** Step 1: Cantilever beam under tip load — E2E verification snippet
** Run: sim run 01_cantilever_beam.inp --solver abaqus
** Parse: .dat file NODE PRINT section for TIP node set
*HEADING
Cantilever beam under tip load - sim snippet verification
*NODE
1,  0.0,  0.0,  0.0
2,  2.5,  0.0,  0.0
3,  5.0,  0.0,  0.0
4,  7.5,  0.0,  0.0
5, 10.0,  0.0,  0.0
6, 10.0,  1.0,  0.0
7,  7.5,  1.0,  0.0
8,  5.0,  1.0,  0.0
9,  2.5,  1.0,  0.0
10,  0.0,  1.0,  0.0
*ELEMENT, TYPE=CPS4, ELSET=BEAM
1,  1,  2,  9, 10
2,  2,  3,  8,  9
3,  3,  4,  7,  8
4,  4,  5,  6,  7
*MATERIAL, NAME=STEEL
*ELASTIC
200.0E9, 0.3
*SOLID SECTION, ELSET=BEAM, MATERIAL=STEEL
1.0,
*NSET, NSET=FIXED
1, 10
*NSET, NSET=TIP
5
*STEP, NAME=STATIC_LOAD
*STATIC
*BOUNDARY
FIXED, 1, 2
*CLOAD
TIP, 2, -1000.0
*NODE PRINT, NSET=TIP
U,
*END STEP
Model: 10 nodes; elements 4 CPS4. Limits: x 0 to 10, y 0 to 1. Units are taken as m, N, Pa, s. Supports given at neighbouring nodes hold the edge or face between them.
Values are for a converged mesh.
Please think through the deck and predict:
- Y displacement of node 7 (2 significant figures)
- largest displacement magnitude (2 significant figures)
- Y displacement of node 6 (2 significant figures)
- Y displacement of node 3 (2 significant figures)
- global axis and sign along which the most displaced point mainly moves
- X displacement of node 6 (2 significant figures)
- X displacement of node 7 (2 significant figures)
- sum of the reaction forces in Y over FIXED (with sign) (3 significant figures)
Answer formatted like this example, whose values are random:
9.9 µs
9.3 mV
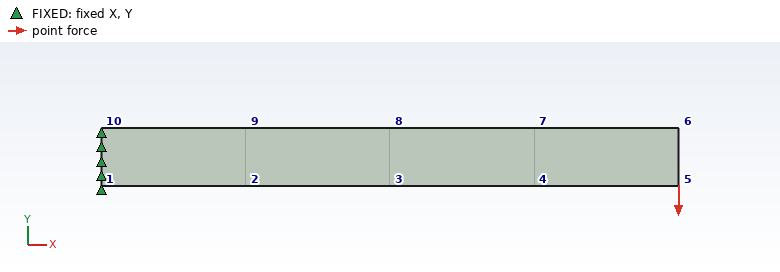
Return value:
-1.2e-05 m
2.0e-05 m
-2.0e-05 m
-6.1e-06 m
-Y
1.5e-06 m
1.4e-06 m
1000 N
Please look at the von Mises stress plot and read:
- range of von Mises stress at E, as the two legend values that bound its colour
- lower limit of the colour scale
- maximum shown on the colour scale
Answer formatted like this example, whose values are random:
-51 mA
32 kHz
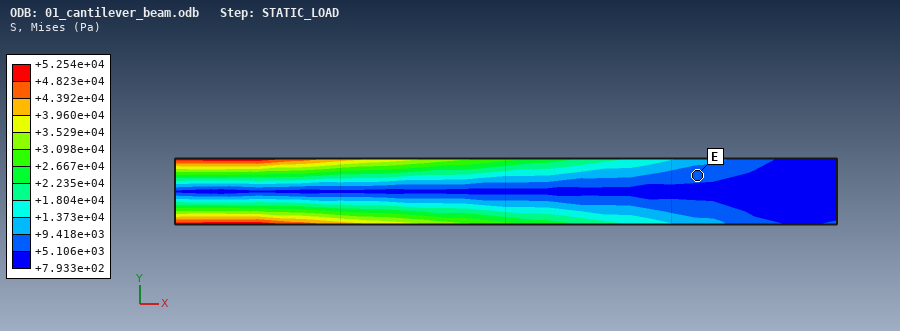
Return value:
+5.106e+03 to +9.418e+03 Pa
+7.933e+02 Pa
+5.254e+04 Pa
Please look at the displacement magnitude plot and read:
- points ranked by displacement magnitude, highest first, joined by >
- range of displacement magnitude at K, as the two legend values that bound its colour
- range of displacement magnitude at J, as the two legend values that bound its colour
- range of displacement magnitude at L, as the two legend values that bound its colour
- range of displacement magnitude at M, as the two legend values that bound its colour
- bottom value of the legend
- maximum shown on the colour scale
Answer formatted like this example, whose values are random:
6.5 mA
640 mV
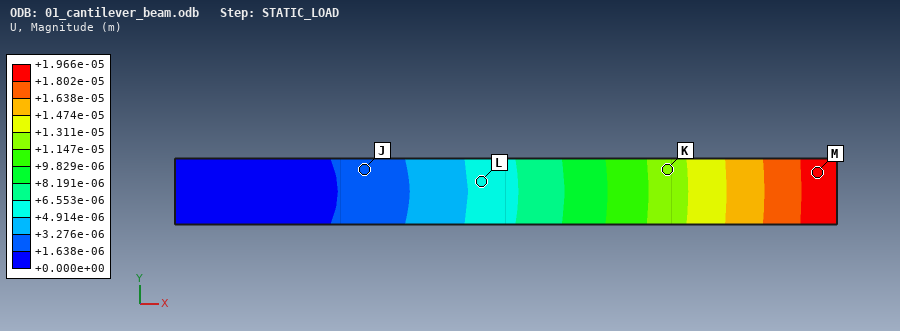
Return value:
M > K > L > J
+1.147e-05 to +1.311e-05 m
+1.638e-06 to +3.276e-06 m
+4.914e-06 to +6.553e-06 m
+1.802e-05 to +1.966e-05 m
+0.000e+00 m
+1.966e-05 m
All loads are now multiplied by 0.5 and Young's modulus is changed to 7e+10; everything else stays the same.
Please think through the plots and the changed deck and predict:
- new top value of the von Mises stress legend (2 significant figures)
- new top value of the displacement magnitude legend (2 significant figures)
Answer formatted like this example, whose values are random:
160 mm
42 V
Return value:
26000 Pa
2.8e-05 m
